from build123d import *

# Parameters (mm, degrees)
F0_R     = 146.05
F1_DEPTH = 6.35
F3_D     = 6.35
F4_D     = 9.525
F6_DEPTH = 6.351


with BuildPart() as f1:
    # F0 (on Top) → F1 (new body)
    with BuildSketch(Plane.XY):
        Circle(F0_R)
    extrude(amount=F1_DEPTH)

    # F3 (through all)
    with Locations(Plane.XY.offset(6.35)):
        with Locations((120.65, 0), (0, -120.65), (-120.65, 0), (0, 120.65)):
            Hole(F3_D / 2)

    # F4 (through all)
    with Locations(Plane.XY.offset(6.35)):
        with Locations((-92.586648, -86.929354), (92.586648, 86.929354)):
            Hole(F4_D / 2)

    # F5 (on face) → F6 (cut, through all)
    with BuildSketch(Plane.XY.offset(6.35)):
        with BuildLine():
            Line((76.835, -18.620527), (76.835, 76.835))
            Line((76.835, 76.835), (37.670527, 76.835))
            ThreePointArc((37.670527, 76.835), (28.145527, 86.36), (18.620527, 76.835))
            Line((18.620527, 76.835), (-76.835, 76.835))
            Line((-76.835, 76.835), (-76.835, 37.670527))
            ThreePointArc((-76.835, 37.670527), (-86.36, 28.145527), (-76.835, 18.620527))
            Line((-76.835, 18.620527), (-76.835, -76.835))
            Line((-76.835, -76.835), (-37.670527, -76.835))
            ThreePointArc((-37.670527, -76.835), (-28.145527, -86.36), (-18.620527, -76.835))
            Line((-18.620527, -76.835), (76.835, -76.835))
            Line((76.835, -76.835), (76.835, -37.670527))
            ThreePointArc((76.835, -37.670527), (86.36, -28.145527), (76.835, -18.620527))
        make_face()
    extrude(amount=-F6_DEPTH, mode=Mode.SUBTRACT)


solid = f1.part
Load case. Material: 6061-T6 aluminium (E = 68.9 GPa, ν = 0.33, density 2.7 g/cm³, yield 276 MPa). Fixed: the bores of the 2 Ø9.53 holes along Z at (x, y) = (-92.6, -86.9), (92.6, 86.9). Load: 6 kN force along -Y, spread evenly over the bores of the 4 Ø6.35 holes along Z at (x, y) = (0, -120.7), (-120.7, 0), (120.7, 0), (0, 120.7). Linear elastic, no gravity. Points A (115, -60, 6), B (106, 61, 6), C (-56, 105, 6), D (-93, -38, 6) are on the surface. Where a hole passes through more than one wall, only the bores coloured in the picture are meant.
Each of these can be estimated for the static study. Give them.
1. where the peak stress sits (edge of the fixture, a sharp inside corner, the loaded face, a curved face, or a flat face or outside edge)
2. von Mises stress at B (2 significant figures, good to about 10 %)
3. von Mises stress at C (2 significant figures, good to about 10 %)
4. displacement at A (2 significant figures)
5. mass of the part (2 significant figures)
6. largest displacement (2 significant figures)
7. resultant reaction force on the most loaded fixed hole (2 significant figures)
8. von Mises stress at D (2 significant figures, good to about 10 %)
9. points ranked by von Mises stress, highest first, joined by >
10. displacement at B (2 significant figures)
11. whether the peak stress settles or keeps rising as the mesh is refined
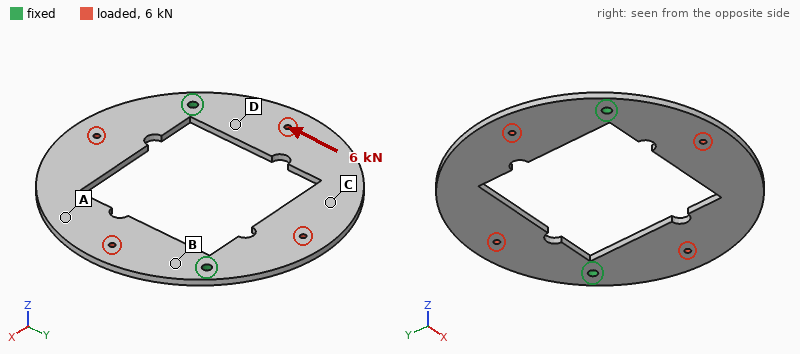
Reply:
edge of the fixture
8.9 MPa
3.8 MPa
20 µm
730 g
32 µm
3.0 kN
6.2 MPa
B > D > C > A
6.9 µm
keeps rising
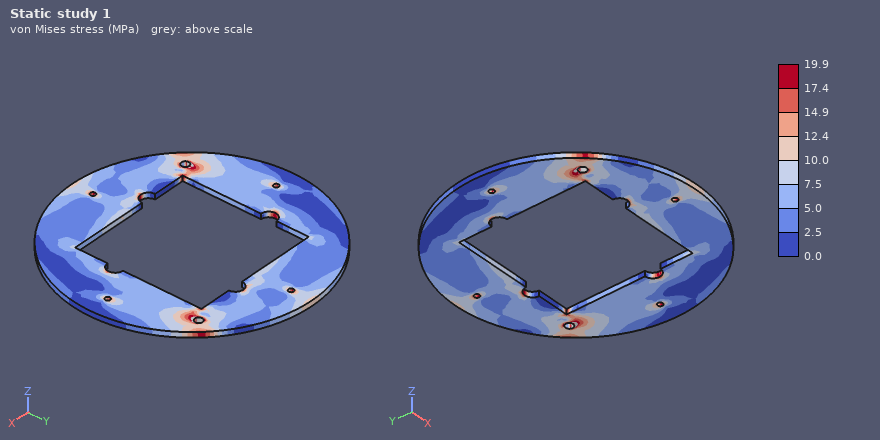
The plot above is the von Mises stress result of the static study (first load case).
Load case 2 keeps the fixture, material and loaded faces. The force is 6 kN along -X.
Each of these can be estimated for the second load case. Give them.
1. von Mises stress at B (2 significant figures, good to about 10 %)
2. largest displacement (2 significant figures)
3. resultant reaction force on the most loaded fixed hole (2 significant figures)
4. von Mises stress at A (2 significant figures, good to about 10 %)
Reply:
6.9 MPa
31 µm
3.0 kN
4.2 MPa
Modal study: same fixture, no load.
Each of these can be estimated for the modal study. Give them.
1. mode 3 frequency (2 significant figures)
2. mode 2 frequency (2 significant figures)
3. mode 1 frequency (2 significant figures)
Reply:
510 Hz
180 Hz
170 Hz
